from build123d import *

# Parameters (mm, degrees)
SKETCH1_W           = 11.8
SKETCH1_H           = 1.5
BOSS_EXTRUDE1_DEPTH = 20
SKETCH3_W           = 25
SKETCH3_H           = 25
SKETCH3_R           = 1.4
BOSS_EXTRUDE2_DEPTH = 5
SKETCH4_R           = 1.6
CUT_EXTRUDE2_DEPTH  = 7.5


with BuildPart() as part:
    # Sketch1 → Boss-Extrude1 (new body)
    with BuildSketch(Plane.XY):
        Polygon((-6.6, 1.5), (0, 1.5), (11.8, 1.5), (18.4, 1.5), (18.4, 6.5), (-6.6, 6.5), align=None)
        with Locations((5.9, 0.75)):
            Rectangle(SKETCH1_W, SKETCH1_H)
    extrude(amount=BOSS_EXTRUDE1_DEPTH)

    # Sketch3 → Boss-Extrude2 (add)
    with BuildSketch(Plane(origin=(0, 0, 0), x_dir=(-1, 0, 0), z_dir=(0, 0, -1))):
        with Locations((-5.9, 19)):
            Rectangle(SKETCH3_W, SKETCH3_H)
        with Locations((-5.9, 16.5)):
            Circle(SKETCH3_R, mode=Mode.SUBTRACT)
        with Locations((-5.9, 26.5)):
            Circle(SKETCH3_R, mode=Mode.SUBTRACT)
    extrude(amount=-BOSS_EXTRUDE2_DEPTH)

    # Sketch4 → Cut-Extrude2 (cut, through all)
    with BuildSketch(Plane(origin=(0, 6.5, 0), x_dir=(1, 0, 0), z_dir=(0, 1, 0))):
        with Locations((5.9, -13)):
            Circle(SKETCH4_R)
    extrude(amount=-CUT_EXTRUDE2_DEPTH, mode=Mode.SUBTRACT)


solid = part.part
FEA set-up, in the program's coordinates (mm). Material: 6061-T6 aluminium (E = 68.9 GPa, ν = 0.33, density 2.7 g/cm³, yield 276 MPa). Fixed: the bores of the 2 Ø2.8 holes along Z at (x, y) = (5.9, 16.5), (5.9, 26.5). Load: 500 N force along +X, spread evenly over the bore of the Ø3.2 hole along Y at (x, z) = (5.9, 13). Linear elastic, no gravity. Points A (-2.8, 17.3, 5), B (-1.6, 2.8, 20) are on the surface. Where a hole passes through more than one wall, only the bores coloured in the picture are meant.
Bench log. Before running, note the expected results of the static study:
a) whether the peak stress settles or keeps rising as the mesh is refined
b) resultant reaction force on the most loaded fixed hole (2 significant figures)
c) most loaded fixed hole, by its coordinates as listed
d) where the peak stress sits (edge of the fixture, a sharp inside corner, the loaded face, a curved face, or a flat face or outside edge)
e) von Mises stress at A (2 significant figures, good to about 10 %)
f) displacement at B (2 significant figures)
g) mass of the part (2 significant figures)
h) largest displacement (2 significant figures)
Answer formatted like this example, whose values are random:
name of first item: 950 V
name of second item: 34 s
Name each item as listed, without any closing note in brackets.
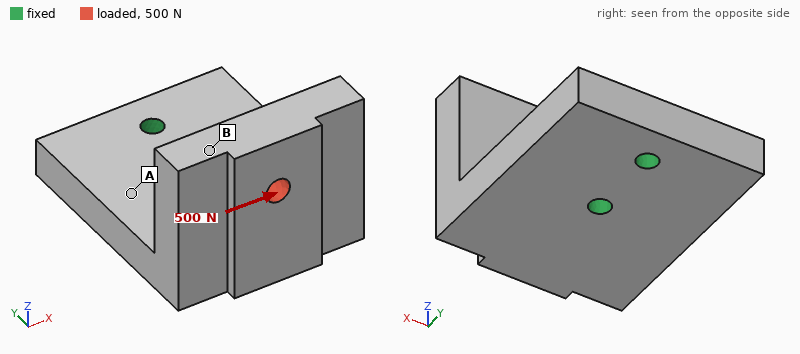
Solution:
whether the peak stress settles or keeps rising as the mesh is refined: keeps rising
resultant reaction force on the most loaded fixed hole: 1000 N
most loaded fixed hole, by its coordinates as listed: (5.9, 16.5)
where the peak stress sits: edge of the fixture
von Mises stress at A: 19 MPa
displacement at B: 56 µm
mass of the part: 16 g
largest displacement: 62 µm
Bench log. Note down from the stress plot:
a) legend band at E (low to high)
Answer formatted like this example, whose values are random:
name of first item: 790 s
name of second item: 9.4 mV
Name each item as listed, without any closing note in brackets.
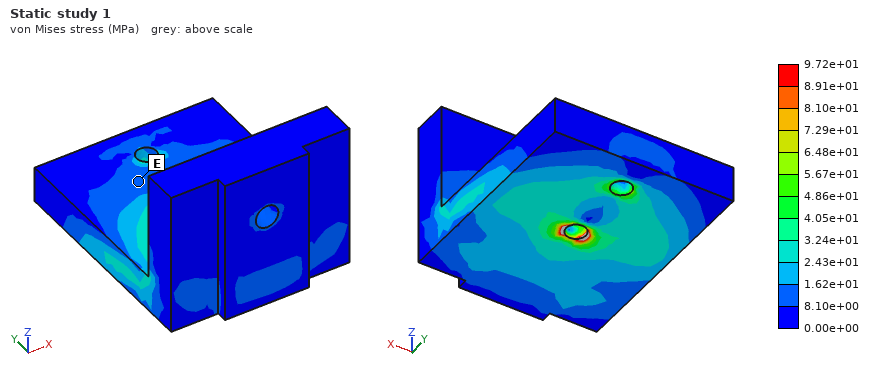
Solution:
legend band at E: 8.10e+00 to 1.62e+01 MPa
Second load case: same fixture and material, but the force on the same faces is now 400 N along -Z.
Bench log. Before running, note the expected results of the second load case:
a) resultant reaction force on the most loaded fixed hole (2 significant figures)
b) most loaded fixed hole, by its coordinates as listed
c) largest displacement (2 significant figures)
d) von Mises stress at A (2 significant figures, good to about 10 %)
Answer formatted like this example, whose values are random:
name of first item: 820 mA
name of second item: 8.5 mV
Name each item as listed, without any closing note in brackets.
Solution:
resultant reaction force on the most loaded fixed hole: 600 N
most loaded fixed hole, by its coordinates as listed: (5.9, 16.5)
largest displacement: 54 µm
von Mises stress at A: 23 MPa
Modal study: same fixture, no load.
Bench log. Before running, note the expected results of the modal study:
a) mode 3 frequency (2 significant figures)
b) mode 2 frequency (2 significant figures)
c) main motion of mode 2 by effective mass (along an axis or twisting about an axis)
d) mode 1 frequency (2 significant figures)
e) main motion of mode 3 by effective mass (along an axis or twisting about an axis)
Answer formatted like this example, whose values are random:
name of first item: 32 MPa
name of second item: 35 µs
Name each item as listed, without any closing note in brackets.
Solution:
mode 3 frequency: 14 kHz
mode 2 frequency: 6500 Hz
main motion of mode 2 by effective mass: along X
mode 1 frequency: 5100 Hz
main motion of mode 3 by effective mass: along Z
